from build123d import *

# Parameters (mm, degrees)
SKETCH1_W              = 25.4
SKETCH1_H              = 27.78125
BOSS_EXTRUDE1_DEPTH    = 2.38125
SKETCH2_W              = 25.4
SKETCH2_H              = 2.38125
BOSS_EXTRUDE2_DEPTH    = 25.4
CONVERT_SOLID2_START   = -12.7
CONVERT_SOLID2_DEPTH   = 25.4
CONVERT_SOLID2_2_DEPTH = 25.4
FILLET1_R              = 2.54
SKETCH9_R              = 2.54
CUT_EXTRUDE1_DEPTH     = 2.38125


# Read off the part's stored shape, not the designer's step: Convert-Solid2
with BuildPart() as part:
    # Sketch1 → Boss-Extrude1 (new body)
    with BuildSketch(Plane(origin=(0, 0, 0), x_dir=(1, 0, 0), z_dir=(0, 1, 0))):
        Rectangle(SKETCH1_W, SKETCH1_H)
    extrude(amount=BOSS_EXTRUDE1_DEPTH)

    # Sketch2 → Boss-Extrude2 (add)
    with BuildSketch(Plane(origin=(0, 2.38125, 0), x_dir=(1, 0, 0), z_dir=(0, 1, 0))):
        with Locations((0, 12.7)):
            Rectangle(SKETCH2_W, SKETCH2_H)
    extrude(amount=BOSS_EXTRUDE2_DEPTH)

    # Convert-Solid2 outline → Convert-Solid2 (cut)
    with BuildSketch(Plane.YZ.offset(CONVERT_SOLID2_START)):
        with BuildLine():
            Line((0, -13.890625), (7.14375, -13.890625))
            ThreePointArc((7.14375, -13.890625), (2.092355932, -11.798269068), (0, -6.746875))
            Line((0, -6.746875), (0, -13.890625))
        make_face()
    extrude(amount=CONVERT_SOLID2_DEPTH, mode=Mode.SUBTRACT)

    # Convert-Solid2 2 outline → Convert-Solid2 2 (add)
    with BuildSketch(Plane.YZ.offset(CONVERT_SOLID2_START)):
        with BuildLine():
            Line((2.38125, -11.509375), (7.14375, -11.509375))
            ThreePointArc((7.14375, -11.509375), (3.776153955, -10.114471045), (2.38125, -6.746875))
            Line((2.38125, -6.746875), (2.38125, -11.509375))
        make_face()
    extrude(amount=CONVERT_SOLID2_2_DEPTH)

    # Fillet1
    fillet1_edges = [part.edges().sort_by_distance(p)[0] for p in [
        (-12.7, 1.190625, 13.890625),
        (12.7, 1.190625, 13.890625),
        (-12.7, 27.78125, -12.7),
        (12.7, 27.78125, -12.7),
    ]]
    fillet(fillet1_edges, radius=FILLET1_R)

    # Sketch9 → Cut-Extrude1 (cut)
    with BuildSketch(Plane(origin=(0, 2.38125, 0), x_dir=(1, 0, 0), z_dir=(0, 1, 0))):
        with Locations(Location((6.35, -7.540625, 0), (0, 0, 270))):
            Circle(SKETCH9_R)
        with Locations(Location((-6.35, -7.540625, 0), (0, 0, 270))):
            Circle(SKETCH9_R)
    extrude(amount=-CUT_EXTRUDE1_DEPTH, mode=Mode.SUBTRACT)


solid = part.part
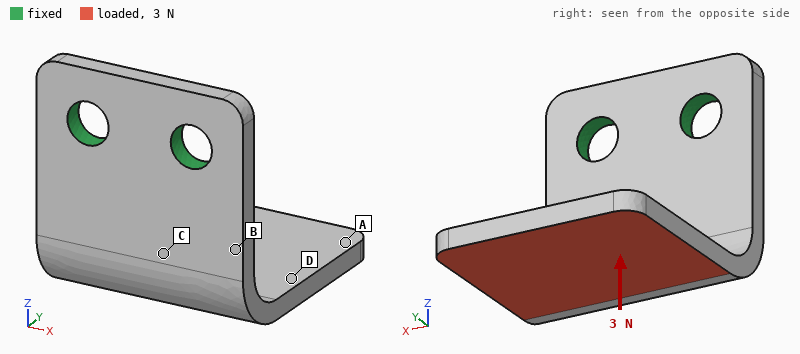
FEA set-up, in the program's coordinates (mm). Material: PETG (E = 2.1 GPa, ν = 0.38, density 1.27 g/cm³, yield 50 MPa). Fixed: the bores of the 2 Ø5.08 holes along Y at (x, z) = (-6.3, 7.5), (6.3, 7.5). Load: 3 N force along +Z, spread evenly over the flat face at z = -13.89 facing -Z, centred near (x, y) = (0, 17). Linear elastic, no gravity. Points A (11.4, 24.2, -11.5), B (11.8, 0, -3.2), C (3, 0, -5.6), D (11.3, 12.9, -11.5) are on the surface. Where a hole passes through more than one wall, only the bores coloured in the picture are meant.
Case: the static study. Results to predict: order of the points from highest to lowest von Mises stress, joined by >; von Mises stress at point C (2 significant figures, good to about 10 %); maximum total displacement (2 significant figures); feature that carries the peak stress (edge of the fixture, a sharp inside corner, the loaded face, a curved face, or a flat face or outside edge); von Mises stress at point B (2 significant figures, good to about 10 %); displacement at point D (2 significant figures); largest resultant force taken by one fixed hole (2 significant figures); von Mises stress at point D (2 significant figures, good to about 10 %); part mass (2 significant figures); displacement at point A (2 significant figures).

B > C > D > A
1.7 MPa
0.47 mm
a flat face or outside edge
2.1 MPa
0.20 mm
1.6 N
0.62 MPa
3.7 g
0.39 mm
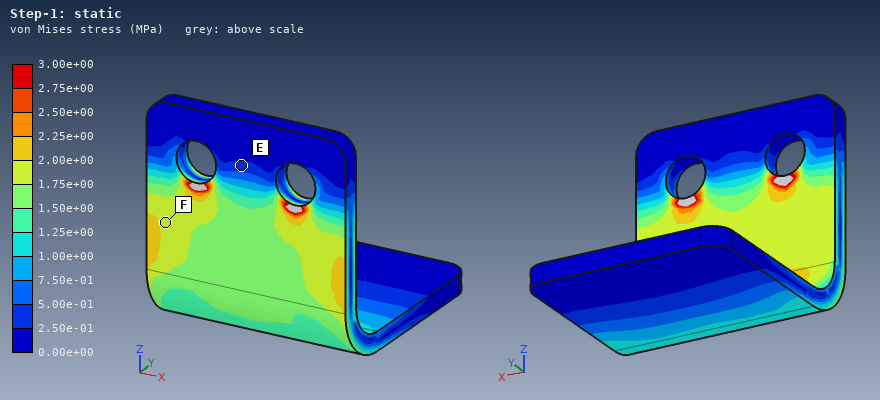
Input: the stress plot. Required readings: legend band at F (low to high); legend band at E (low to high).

1.75e+00 to 2.00e+00 MPa
2.50e-01 to 5.00e-01 MPa
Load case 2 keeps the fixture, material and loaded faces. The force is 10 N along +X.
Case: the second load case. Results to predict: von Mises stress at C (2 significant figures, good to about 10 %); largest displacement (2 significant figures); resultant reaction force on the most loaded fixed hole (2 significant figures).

3.5 MPa
0.53 mm
17 N
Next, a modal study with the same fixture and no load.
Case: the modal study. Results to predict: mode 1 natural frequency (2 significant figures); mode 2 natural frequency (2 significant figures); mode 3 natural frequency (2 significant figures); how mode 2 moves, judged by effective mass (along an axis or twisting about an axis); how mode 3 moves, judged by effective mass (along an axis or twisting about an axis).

350 Hz
600 Hz
1100 Hz
along X
along Y
